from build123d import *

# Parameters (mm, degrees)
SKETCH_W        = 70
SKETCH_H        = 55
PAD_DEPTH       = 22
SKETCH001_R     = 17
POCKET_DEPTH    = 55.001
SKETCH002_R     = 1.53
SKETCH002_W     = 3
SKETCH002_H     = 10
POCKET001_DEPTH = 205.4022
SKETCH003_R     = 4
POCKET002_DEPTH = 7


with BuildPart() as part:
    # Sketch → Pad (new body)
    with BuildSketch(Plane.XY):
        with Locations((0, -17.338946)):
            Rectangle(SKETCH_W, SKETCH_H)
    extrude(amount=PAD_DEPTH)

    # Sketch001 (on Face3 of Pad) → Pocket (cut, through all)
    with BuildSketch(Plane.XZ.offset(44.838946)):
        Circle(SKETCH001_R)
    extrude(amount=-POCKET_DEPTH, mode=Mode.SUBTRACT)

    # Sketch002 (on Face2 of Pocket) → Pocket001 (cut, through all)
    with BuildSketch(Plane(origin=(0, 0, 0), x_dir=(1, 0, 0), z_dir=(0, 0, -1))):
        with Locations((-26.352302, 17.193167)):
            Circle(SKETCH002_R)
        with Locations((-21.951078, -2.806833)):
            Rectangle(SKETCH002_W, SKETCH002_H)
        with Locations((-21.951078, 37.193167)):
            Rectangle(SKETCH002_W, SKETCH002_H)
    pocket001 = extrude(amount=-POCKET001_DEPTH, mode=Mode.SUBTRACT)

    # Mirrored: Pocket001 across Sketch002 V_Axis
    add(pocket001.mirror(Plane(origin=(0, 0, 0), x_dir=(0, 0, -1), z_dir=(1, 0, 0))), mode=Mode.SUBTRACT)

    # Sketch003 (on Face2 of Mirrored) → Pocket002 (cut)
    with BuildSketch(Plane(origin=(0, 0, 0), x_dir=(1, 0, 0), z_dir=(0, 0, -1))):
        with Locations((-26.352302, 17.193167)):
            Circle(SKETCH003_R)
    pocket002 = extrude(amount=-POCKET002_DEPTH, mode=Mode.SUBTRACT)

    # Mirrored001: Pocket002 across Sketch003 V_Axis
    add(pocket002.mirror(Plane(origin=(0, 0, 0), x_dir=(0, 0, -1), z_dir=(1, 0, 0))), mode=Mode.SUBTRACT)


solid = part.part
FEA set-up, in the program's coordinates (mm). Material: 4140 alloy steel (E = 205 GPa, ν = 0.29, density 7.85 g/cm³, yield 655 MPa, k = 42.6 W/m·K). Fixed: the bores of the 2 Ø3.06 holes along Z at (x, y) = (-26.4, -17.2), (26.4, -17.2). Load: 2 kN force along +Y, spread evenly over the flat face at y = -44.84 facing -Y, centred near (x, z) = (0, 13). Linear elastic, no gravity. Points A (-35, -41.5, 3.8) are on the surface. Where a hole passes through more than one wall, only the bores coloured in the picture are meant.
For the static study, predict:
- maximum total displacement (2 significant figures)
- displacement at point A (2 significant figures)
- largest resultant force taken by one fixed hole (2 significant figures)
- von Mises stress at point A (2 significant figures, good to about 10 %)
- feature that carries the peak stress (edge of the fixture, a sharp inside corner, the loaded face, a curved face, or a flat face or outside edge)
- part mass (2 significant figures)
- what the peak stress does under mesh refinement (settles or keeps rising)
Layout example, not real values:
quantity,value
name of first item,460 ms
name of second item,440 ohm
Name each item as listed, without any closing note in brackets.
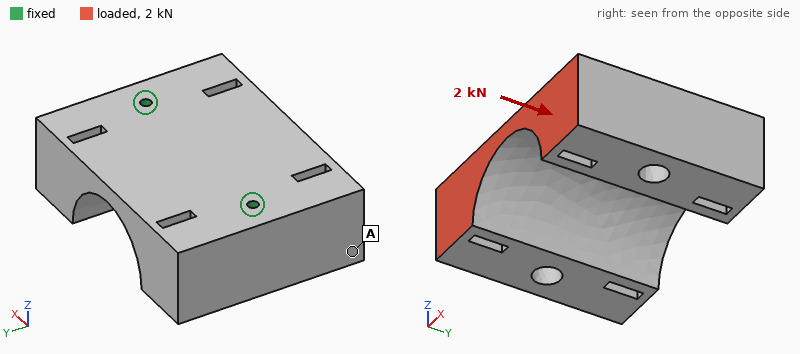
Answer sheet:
quantity,value
maximum total displacement,0.76 µm
displacement at point A,0.58 µm
largest resultant force taken by one fixed hole,1.0 kN
von Mises stress at point A,1.8 MPa
feature that carries the peak stress,edge of the fixture
part mass,440 g
what the peak stress does under mesh refinement,keeps rising
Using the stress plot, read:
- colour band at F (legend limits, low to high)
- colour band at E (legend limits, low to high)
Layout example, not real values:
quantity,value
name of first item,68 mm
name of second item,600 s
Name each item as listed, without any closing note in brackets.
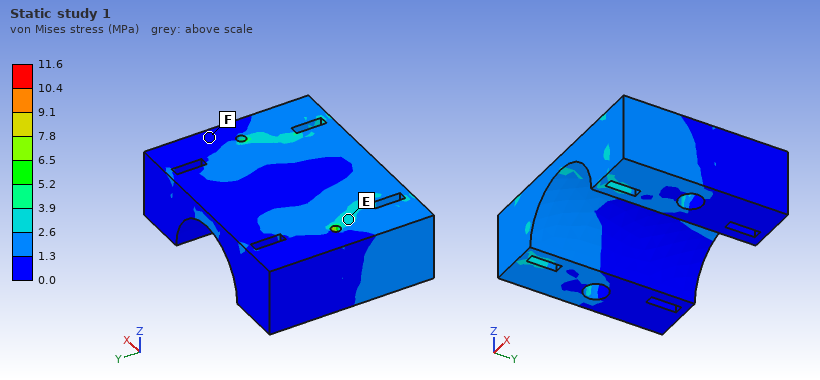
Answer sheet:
quantity,value
colour band at F,0.0 to 1.3 MPa
colour band at E,2.6 to 3.9 MPa
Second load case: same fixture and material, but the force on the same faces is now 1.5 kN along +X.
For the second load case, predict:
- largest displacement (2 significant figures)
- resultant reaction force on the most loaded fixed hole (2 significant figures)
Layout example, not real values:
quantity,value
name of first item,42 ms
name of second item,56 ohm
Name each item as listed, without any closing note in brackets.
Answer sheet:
quantity,value
largest displacement,2.3 µm
resultant reaction force on the most loaded fixed hole,1.1 kN
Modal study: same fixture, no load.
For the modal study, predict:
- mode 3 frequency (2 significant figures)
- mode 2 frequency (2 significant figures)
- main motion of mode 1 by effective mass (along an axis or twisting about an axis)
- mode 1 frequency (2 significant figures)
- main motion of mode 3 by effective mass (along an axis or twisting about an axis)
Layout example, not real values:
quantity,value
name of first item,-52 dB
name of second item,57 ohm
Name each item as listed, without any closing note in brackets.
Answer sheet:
quantity,value
mode 3 frequency,11 kHz
mode 2 frequency,9500 Hz
main motion of mode 1 by effective mass,twisting about X
mode 1 frequency,7600 Hz
main motion of mode 3 by effective mass,along Z
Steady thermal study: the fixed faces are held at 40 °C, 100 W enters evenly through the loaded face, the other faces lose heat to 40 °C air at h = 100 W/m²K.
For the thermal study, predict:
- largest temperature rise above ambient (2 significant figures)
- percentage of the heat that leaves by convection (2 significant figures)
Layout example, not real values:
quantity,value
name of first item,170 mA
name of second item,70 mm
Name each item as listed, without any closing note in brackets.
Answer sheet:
quantity,value
largest temperature rise above ambient,67 K
percentage of the heat that leaves by convection,33 %
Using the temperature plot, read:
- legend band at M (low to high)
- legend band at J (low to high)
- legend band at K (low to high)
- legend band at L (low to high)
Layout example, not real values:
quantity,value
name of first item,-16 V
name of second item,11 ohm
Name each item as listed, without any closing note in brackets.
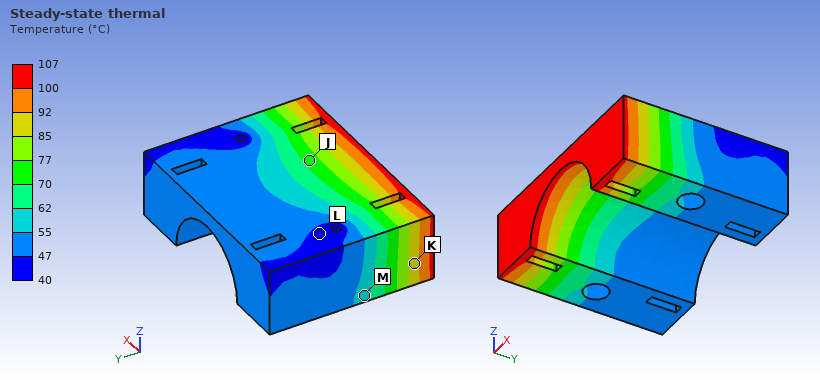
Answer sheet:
quantity,value
legend band at M,55 to 62 °C
legend band at J,70 to 77 °C
legend band at K,85 to 92 °C
legend band at L,40 to 47 °C
